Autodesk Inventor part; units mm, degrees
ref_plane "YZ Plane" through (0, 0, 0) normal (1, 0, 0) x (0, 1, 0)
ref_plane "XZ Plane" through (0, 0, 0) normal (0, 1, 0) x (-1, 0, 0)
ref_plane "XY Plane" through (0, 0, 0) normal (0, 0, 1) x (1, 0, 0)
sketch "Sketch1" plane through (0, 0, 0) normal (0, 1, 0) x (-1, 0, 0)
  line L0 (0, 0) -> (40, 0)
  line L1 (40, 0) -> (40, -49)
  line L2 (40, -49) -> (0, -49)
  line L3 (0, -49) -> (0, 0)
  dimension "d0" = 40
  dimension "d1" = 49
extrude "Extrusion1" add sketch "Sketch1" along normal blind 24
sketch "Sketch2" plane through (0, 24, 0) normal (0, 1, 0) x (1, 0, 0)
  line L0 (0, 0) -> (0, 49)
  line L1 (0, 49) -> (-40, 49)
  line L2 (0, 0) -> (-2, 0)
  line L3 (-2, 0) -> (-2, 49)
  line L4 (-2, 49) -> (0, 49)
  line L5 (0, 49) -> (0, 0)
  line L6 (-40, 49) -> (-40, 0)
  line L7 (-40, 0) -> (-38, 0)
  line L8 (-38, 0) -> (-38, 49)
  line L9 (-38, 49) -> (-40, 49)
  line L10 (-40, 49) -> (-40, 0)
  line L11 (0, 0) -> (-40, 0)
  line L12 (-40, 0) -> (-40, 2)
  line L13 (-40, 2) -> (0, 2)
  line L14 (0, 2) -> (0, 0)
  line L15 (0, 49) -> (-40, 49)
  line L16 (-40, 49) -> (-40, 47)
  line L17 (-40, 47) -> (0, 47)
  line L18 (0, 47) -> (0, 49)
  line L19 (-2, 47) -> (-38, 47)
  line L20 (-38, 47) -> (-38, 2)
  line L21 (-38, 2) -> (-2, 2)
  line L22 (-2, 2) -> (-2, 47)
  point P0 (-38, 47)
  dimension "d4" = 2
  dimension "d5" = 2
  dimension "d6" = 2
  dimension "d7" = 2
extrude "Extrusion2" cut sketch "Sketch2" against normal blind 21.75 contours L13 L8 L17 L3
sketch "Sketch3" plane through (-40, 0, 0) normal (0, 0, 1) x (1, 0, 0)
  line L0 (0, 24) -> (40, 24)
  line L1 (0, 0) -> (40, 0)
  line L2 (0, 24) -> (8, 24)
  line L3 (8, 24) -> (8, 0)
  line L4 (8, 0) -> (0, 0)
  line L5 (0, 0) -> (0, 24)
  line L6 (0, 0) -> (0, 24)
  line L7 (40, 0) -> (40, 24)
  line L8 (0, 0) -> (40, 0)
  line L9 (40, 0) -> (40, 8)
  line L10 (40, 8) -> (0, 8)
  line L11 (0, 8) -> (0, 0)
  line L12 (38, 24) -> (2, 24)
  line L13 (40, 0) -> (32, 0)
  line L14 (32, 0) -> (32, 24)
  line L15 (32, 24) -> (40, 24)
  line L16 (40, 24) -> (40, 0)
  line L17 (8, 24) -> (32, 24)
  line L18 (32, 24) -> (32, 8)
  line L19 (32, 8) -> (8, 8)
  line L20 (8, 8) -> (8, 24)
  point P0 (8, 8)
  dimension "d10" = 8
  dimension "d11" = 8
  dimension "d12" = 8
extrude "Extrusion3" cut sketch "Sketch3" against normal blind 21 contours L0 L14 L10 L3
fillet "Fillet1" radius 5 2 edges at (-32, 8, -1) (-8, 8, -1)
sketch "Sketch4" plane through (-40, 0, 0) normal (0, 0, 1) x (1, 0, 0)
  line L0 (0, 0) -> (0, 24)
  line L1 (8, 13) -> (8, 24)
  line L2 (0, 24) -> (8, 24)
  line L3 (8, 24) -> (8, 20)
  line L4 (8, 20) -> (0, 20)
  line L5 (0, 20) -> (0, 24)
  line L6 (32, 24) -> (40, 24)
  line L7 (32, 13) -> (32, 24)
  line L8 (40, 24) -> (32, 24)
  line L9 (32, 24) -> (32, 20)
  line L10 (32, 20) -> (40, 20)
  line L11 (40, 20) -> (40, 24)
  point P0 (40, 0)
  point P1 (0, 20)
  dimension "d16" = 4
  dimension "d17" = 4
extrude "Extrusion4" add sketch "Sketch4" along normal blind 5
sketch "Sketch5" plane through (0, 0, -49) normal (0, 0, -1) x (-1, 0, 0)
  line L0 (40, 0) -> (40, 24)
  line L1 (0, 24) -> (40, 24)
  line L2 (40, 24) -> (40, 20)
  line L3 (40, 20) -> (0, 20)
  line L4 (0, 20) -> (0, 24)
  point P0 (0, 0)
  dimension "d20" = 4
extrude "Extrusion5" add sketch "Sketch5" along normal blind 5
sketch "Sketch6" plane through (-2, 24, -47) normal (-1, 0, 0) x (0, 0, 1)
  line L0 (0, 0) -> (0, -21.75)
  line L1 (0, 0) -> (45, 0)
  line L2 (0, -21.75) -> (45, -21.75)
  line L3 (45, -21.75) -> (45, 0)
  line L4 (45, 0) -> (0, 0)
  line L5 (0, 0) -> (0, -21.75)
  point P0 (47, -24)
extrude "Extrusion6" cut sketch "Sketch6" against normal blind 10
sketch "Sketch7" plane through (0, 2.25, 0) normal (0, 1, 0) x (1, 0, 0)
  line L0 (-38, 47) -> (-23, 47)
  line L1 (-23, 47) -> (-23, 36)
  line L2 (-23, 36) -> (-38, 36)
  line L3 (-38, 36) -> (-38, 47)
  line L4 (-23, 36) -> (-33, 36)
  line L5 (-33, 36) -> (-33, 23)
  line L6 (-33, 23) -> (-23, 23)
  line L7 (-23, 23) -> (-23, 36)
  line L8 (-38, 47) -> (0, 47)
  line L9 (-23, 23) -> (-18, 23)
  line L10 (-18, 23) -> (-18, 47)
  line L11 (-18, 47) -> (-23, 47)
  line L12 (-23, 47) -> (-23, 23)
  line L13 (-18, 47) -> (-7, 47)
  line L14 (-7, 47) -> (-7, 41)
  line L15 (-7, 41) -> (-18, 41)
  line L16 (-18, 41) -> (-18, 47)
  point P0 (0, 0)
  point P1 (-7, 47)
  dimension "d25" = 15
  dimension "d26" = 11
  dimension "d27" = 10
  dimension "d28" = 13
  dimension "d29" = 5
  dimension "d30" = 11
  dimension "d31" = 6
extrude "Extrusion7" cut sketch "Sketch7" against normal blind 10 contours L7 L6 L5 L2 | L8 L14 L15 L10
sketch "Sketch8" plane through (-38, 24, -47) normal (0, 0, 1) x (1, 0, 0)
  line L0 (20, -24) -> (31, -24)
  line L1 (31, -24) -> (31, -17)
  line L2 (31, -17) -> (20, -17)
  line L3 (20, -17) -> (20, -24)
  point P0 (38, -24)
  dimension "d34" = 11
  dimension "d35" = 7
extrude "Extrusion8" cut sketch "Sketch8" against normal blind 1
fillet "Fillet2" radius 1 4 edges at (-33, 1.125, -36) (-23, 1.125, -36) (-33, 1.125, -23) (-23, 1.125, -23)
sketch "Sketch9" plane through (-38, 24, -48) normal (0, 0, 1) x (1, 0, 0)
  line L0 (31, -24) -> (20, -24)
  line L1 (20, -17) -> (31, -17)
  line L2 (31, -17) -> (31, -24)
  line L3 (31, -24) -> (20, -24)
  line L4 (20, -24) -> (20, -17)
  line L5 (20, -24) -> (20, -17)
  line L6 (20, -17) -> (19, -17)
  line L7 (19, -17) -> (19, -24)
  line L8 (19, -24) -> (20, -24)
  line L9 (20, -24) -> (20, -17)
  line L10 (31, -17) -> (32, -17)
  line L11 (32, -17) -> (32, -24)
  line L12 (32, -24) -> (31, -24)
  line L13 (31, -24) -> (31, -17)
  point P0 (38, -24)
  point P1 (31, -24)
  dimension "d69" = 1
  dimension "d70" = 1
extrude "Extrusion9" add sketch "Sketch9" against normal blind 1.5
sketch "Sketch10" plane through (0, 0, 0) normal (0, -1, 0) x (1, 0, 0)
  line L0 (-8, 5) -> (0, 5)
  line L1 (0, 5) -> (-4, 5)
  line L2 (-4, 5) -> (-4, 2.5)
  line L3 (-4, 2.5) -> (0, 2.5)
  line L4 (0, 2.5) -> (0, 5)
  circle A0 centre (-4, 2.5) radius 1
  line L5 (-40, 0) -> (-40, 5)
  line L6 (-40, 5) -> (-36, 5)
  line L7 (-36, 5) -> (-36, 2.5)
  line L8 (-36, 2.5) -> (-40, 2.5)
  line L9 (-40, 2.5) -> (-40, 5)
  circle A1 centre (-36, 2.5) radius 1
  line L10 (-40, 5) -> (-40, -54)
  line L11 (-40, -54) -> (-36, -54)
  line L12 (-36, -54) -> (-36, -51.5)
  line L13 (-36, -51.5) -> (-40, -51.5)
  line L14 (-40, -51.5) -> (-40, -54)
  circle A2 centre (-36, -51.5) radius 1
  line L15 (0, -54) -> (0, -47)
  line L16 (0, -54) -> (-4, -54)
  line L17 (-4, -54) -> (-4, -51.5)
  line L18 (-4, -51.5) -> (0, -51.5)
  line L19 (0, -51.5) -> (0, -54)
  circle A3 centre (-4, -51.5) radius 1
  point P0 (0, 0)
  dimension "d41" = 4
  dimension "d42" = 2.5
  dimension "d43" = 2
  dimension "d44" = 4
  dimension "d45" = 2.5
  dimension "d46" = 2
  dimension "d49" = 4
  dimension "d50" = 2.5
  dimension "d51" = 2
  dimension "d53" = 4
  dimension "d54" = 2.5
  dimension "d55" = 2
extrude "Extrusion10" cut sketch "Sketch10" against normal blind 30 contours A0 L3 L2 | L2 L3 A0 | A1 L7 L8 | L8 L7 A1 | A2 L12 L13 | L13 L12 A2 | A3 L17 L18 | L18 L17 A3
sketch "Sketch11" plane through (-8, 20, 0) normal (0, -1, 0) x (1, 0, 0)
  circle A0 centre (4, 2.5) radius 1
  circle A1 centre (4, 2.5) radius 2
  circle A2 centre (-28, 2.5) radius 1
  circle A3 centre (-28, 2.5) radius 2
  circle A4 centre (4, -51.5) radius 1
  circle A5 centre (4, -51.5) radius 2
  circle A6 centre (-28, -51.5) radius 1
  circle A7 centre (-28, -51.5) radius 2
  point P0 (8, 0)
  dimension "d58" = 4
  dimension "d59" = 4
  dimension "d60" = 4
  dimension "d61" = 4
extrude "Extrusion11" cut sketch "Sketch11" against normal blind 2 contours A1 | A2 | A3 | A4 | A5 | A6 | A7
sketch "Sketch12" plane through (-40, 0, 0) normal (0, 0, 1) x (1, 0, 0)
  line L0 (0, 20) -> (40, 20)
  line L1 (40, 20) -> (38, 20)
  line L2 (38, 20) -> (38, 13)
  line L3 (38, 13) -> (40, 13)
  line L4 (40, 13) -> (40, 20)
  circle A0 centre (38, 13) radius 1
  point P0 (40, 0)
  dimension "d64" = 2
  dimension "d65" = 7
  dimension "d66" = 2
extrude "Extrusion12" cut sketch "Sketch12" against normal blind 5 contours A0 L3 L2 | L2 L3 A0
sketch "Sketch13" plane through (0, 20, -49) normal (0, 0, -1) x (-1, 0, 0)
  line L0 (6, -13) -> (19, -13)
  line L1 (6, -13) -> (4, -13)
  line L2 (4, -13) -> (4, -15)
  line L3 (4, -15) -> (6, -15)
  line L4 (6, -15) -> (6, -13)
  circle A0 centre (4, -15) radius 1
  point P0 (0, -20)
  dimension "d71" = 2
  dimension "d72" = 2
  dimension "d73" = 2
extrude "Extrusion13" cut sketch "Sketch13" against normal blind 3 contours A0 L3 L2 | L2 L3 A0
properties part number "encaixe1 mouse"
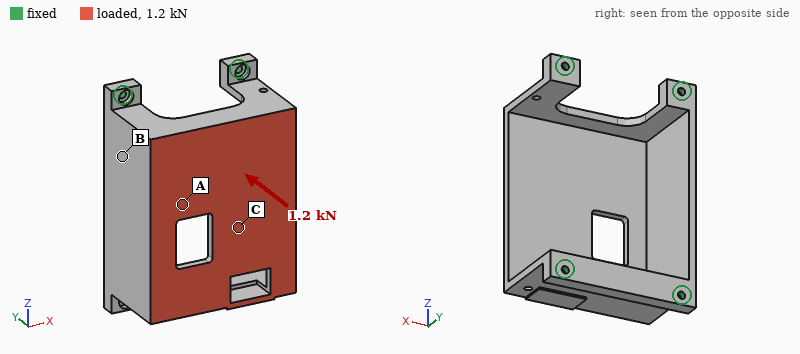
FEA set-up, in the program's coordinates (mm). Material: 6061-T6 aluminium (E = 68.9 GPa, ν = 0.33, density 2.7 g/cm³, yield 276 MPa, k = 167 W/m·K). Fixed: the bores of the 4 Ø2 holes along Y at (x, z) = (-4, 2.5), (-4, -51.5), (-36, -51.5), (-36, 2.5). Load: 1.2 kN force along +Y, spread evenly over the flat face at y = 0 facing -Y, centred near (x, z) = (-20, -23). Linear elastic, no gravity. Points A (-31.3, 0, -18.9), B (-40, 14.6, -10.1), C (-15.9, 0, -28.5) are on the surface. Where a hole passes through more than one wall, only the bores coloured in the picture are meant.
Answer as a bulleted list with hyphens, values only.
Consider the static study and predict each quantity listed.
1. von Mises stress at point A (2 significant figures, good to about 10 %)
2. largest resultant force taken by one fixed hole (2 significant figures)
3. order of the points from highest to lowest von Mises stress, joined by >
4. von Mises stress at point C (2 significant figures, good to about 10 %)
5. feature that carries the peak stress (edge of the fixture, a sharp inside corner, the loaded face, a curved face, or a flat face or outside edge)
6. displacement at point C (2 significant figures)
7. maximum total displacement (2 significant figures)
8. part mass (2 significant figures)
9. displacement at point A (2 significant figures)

- 43 MPa
- 350 N
- C > A > B
- 73 MPa
- a curved face
- 0.18 mm
- 0.27 mm
- 26 g
- 0.068 mm
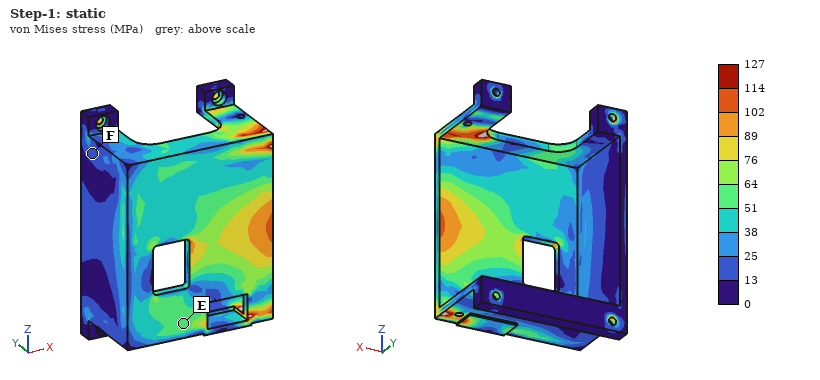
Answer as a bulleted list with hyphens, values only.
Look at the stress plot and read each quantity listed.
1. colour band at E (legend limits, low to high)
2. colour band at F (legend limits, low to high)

- 51 to 64 MPa
- 13 to 25 MPa
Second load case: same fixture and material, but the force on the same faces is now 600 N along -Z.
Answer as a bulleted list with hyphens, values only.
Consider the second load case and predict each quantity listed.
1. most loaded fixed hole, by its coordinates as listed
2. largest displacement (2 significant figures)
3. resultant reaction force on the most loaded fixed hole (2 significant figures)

- (-36, -51.5)
- 73 µm
- 510 N
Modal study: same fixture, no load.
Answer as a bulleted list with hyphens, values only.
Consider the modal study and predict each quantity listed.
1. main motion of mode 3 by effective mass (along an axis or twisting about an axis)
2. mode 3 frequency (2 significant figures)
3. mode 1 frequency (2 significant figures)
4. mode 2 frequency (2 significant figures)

- along X
- 5800 Hz
- 4100 Hz
- 4200 Hz
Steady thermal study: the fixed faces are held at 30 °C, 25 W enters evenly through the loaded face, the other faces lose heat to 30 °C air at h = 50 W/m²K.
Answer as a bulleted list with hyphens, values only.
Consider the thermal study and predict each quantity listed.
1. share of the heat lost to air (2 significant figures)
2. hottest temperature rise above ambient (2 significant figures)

- 26 %
- 32 K
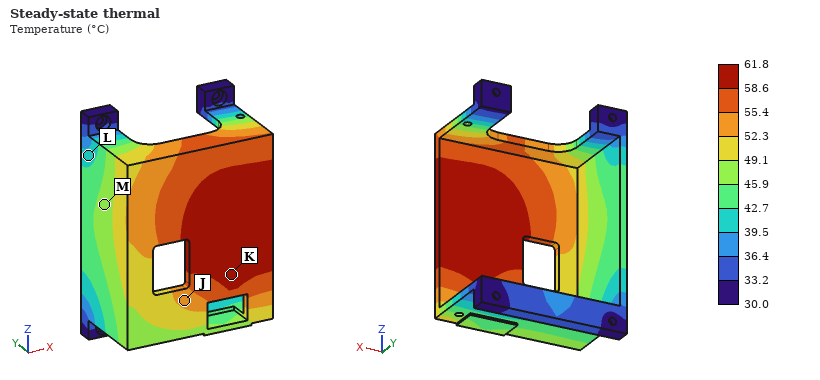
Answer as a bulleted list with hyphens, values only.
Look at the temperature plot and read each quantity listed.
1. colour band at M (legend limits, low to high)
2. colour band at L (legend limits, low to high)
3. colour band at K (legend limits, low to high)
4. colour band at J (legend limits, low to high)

- 45.9 to 49.1 °C
- 39.5 to 42.7 °C
- 58.6 to 61.8 °C
- 52.3 to 55.4 °C
